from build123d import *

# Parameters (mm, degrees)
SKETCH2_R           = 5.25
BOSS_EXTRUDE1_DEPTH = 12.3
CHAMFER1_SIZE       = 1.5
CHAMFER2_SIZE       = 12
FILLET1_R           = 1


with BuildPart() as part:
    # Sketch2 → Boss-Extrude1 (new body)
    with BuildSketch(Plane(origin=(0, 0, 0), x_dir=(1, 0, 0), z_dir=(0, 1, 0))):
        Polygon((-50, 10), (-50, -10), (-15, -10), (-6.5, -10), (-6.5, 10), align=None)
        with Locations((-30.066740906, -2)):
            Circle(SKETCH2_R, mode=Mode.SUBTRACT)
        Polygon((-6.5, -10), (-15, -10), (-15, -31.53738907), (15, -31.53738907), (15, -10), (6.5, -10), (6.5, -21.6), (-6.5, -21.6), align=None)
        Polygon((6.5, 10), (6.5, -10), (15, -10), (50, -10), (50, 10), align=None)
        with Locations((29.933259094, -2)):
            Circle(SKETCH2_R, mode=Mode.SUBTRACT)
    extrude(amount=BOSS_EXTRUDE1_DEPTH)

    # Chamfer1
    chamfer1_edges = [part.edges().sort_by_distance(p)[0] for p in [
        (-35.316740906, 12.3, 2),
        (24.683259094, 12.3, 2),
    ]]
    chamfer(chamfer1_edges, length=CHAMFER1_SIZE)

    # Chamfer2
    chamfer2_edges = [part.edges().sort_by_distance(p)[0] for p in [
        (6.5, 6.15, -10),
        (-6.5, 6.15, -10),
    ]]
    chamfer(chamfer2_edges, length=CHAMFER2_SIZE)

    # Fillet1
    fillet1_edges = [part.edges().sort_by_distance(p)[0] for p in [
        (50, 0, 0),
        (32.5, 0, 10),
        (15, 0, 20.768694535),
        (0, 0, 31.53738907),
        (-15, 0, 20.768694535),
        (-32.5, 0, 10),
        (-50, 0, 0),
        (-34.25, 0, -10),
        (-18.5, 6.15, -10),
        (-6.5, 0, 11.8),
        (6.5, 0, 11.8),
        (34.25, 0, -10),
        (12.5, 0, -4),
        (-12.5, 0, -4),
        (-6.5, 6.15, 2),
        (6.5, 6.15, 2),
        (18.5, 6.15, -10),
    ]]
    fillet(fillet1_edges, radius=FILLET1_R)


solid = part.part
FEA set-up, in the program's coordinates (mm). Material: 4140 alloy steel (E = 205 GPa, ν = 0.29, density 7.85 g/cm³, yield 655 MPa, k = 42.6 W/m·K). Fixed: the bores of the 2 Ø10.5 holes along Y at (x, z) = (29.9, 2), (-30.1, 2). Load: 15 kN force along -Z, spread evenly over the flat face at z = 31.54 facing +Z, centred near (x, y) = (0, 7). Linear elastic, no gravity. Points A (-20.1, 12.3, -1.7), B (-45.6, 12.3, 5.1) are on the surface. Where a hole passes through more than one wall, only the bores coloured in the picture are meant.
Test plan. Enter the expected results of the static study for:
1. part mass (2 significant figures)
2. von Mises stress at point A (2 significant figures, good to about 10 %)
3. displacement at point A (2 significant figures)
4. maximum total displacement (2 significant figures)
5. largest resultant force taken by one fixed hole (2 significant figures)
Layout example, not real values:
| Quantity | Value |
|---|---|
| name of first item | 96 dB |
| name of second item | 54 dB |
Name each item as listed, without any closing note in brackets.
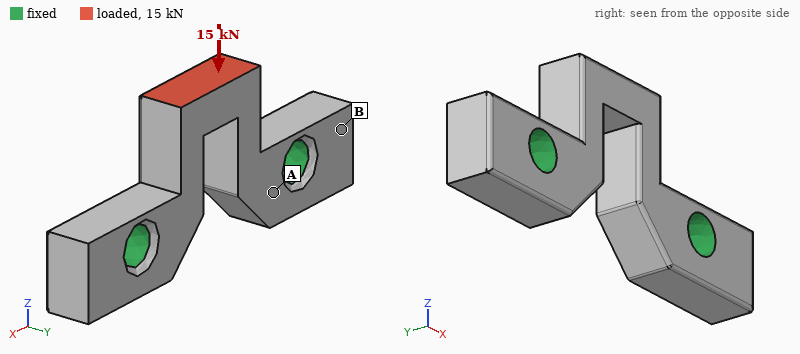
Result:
| Quantity | Value |
|---|---|
| part mass | 180 g |
| von Mises stress at point A | 70 MPa |
| displacement at point A | 5.8 µm |
| maximum total displacement | 27 µm |
| largest resultant force taken by one fixed hole | 7.8 kN |
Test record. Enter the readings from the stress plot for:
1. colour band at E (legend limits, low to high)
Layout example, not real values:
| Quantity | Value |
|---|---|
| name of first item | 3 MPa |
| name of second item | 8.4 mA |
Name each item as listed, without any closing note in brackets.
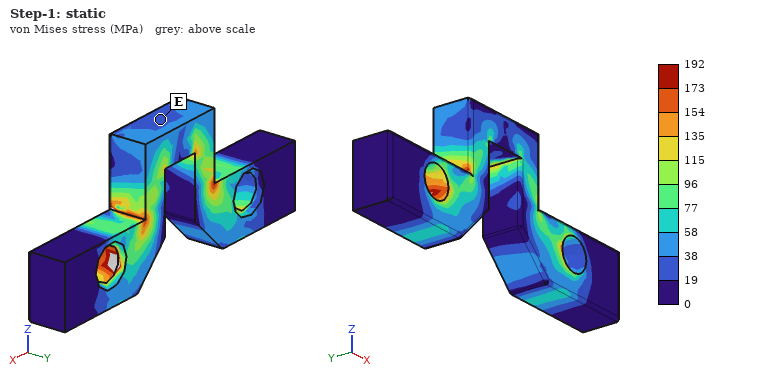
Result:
| Quantity | Value |
|---|---|
| colour band at E | 19 to 38 MPa |
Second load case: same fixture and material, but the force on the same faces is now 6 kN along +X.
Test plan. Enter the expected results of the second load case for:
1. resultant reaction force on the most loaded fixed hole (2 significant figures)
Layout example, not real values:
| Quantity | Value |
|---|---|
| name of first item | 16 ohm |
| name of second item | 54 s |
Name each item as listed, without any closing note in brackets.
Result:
| Quantity | Value |
|---|---|
| resultant reaction force on the most loaded fixed hole | 5.0 kN |
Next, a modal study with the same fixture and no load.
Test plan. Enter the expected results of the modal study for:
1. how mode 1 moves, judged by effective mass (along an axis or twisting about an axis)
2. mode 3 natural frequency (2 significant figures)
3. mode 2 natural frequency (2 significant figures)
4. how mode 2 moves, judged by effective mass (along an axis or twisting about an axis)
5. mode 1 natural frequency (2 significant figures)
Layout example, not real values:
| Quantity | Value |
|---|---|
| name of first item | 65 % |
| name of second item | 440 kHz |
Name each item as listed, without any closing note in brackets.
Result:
| Quantity | Value |
|---|---|
| how mode 1 moves, judged by effective mass | along Y |
| mode 3 natural frequency | 14 kHz |
| mode 2 natural frequency | 13 kHz |
| how mode 2 moves, judged by effective mass | along X |
| mode 1 natural frequency | 6300 Hz |
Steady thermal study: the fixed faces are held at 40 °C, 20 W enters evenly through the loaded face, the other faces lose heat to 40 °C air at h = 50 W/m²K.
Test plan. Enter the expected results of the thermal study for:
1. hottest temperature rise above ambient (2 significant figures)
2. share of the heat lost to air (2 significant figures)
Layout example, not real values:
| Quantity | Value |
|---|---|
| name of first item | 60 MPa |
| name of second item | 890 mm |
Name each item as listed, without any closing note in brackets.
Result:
| Quantity | Value |
|---|---|
| hottest temperature rise above ambient | 58 K |
| share of the heat lost to air | 24 % |
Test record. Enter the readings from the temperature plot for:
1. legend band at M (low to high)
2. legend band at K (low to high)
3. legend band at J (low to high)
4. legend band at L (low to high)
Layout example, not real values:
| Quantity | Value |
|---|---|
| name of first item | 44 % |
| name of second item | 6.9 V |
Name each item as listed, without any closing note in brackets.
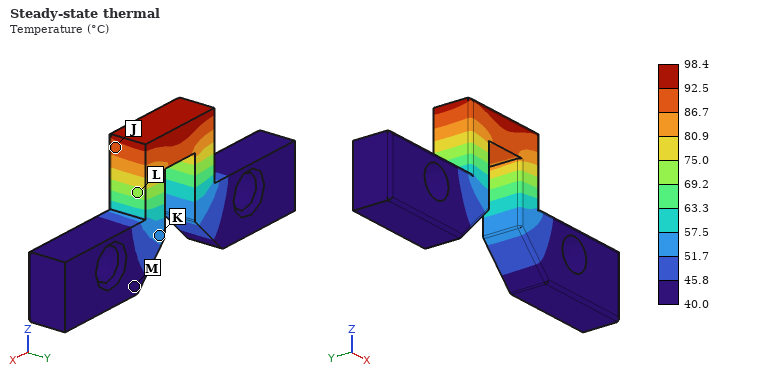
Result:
| Quantity | Value |
|---|---|
| legend band at M | 40.0 to 45.8 °C |
| legend band at K | 51.7 to 57.5 °C |
| legend band at J | 86.7 to 92.5 °C |
| legend band at L | 69.2 to 75.0 °C |
